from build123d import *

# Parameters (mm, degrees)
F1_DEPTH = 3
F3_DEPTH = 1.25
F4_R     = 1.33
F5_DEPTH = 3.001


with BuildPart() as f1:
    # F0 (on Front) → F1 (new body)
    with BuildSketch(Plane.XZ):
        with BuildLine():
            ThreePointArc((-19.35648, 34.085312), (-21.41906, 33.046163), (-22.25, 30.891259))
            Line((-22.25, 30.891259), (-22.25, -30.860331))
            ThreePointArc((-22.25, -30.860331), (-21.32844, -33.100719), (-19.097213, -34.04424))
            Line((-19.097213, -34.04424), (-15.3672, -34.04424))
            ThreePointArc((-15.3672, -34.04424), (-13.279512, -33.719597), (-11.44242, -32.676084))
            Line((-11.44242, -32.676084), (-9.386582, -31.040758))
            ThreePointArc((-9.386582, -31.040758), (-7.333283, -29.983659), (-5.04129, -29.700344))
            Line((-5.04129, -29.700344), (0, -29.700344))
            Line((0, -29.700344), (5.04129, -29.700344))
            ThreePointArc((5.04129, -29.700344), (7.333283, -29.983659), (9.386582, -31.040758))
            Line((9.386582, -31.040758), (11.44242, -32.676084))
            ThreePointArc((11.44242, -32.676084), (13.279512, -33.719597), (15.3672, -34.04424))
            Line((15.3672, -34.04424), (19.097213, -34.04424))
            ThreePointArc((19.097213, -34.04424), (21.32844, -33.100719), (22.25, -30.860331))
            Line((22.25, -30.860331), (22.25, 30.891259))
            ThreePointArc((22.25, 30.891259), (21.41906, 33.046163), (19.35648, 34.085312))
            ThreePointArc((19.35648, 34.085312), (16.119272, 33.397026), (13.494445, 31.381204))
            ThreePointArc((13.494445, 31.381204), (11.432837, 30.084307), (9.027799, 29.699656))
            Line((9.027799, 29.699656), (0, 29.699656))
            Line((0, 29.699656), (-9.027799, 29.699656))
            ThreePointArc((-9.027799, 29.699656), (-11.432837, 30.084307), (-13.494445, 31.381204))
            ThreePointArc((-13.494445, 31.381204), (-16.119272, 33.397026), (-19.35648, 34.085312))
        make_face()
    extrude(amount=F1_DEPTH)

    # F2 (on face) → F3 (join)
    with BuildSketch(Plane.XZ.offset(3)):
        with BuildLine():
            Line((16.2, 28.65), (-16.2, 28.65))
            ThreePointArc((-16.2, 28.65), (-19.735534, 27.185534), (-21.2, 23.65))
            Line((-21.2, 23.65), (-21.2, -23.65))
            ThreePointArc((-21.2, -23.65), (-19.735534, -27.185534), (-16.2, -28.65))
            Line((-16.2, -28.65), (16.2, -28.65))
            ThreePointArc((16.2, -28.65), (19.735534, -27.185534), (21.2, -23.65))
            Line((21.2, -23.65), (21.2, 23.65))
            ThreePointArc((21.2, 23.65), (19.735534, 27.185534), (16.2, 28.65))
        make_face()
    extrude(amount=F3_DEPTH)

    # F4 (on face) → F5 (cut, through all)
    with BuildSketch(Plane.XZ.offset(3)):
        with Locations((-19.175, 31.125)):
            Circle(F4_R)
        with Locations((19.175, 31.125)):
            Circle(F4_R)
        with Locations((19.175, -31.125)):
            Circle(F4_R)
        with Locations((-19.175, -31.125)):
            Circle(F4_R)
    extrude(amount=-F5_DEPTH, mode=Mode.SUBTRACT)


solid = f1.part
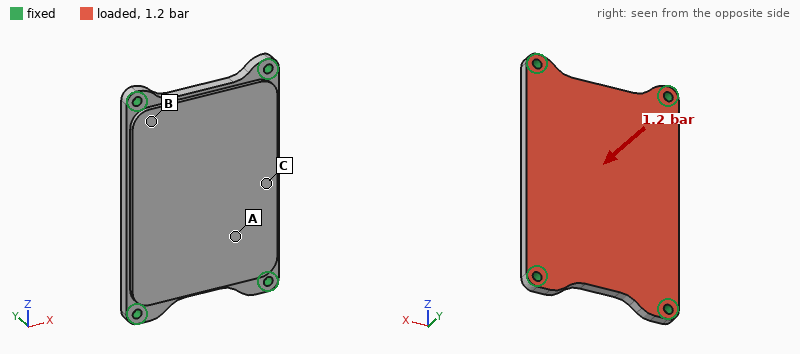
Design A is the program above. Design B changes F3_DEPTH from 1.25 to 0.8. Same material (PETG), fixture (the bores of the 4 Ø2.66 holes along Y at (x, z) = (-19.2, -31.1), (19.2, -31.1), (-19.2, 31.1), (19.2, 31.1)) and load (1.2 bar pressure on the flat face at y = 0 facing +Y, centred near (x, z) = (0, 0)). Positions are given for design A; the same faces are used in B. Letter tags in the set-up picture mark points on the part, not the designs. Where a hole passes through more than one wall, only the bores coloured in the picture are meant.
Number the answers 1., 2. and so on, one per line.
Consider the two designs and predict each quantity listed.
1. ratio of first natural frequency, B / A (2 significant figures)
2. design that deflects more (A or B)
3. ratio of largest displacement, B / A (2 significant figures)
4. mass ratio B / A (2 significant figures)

1. 0.95
2. B
3. 1.2
4. 0.90
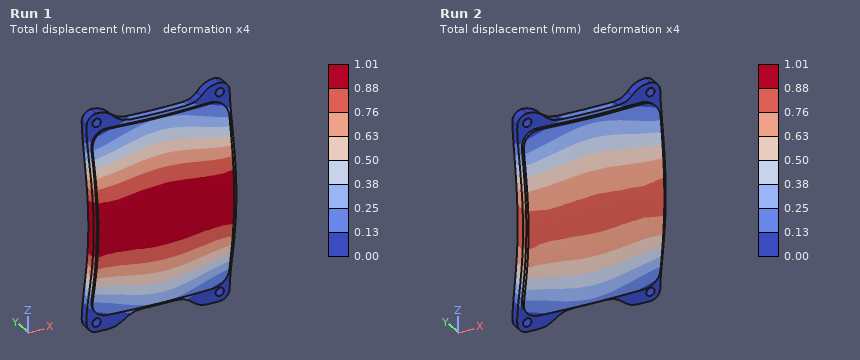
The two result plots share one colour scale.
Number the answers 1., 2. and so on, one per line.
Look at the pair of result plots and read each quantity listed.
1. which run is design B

1. Run 1
